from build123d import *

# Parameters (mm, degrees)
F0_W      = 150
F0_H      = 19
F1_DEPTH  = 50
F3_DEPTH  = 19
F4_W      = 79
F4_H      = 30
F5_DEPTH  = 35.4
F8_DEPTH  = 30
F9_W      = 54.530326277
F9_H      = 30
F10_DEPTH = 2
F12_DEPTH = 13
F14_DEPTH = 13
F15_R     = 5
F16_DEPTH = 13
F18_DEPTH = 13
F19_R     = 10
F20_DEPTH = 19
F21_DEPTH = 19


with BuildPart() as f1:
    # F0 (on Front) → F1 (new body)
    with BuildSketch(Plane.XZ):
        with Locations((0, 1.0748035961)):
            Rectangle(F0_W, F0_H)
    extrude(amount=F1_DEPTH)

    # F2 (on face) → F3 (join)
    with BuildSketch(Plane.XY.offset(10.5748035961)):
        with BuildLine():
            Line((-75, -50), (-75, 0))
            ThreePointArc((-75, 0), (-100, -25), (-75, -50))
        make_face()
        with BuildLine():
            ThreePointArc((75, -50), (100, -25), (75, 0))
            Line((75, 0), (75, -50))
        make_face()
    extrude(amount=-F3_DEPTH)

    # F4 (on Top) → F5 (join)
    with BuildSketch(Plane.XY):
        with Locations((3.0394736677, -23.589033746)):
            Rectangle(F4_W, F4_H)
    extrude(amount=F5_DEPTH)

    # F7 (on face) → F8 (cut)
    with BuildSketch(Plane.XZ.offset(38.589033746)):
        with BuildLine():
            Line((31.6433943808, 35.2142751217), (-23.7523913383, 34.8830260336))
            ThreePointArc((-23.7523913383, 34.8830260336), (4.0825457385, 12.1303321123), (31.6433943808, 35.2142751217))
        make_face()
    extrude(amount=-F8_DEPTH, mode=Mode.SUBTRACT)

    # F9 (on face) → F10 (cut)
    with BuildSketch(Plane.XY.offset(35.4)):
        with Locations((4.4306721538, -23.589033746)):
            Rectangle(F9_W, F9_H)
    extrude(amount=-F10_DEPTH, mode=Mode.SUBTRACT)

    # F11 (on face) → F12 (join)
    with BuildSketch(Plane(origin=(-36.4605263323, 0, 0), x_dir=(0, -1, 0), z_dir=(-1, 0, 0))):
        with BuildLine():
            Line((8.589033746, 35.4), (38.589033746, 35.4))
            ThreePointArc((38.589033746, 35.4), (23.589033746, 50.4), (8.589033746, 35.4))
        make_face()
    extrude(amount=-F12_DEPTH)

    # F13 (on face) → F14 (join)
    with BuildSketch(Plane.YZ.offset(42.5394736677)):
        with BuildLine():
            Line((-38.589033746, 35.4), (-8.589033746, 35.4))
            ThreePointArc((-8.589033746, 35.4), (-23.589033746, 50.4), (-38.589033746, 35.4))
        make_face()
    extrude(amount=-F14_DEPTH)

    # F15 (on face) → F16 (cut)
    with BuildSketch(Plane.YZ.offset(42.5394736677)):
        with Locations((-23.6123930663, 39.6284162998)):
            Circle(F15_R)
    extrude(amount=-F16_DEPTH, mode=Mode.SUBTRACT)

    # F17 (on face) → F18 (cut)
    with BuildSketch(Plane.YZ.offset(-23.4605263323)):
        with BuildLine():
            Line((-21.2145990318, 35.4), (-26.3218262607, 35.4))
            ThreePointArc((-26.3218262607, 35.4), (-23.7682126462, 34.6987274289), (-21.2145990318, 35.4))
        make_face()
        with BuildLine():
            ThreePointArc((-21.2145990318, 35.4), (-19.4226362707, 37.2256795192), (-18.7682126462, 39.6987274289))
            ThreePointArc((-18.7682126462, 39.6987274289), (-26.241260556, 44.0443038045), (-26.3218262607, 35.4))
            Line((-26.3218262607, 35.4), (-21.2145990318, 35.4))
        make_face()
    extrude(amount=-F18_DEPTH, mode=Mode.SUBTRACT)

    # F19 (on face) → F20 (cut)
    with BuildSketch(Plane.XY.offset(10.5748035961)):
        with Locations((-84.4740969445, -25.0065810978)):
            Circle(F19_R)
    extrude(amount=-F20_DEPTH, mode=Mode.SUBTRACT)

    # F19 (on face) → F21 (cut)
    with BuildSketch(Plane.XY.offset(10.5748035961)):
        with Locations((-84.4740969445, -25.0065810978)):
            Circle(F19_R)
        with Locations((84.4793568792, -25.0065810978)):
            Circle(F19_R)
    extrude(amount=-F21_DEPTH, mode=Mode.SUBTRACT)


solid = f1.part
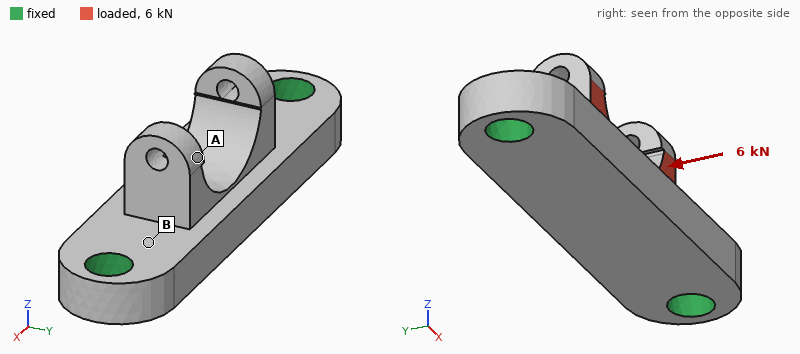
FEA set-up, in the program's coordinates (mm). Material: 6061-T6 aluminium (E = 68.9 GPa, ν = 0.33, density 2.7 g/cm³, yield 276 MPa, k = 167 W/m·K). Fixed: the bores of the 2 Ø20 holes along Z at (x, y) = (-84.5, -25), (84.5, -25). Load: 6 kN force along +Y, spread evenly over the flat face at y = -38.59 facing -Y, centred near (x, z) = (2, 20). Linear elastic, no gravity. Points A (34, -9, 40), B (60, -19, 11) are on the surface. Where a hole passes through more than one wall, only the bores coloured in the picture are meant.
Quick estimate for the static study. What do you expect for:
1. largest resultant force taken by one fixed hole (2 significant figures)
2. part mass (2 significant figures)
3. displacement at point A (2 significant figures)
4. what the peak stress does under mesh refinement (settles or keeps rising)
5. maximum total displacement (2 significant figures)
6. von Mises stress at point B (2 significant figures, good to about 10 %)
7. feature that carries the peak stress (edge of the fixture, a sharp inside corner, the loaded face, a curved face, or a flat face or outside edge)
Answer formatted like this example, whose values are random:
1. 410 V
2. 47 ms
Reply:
1. 3.1 kN
2. 550 g
3. 59 µm
4. keeps rising
5. 73 µm
6. 23 MPa
7. edge of the fixture
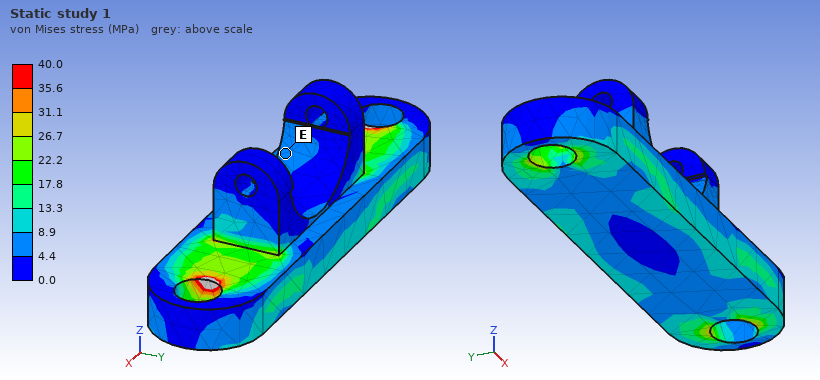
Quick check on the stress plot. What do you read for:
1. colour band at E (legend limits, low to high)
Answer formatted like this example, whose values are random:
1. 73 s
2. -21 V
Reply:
1. 4.4 to 8.9 MPa
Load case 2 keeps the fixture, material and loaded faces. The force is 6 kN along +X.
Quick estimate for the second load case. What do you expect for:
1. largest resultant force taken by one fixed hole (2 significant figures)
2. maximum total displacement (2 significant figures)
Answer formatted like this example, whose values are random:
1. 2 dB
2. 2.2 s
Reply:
1. 3.3 kN
2. 20 µm
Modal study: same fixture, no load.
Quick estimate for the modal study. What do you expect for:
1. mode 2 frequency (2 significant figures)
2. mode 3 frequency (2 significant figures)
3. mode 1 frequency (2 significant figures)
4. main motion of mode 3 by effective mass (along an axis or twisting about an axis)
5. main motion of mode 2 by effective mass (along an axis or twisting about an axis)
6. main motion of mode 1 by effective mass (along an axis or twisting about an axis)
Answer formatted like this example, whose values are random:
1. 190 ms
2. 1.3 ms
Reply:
1. 4100 Hz
2. 5700 Hz
3. 3300 Hz
4. along Y
5. along Y
6. along Z
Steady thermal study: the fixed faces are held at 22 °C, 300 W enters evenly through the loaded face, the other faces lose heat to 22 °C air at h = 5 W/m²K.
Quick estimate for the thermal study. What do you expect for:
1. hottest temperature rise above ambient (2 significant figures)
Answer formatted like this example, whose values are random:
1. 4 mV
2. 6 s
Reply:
1. 79 K
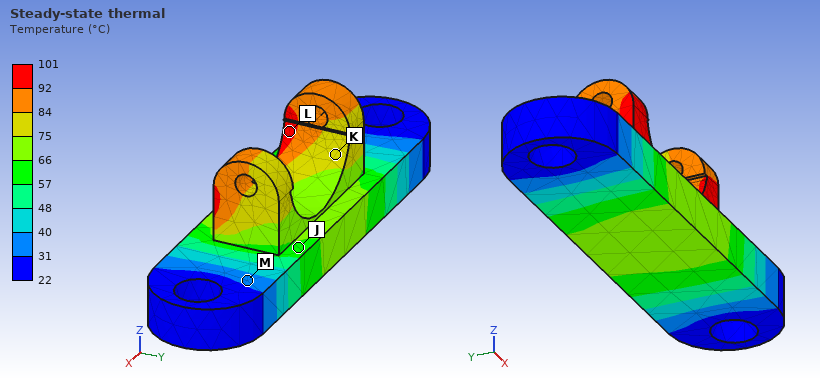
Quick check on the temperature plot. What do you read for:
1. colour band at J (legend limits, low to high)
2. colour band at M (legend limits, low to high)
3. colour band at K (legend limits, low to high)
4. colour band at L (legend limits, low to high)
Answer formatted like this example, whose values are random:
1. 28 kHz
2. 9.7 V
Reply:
1. 57 to 66 °C
2. 31 to 40 °C
3. 75 to 84 °C
4. 92 to 101 °C
